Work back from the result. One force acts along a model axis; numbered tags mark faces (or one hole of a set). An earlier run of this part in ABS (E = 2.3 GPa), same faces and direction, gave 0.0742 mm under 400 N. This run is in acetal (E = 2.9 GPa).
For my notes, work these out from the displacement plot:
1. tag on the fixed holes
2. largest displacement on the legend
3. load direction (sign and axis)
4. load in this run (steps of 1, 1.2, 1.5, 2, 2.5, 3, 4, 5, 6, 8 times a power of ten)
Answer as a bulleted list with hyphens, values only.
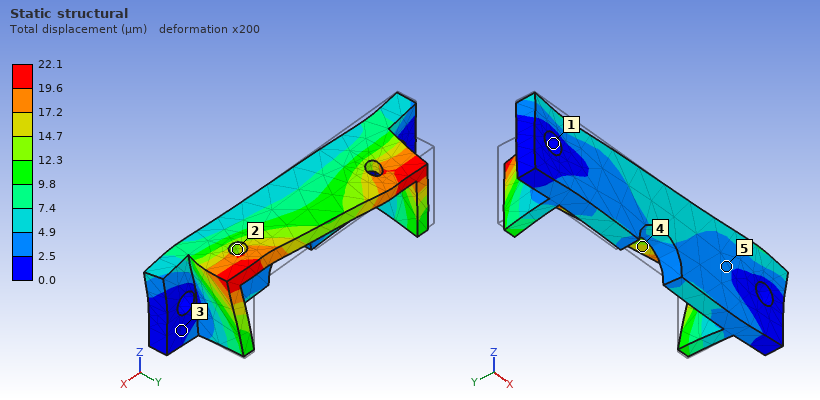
- 1
- 22.1 µm
- +X
- 150 N
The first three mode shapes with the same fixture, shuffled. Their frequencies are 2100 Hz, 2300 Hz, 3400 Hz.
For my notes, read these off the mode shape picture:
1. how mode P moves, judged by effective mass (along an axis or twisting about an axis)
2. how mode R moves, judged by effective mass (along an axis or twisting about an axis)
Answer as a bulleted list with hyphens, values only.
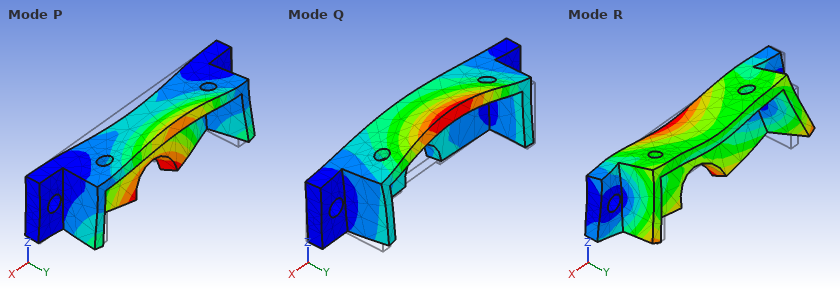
- along Y
- along Z
